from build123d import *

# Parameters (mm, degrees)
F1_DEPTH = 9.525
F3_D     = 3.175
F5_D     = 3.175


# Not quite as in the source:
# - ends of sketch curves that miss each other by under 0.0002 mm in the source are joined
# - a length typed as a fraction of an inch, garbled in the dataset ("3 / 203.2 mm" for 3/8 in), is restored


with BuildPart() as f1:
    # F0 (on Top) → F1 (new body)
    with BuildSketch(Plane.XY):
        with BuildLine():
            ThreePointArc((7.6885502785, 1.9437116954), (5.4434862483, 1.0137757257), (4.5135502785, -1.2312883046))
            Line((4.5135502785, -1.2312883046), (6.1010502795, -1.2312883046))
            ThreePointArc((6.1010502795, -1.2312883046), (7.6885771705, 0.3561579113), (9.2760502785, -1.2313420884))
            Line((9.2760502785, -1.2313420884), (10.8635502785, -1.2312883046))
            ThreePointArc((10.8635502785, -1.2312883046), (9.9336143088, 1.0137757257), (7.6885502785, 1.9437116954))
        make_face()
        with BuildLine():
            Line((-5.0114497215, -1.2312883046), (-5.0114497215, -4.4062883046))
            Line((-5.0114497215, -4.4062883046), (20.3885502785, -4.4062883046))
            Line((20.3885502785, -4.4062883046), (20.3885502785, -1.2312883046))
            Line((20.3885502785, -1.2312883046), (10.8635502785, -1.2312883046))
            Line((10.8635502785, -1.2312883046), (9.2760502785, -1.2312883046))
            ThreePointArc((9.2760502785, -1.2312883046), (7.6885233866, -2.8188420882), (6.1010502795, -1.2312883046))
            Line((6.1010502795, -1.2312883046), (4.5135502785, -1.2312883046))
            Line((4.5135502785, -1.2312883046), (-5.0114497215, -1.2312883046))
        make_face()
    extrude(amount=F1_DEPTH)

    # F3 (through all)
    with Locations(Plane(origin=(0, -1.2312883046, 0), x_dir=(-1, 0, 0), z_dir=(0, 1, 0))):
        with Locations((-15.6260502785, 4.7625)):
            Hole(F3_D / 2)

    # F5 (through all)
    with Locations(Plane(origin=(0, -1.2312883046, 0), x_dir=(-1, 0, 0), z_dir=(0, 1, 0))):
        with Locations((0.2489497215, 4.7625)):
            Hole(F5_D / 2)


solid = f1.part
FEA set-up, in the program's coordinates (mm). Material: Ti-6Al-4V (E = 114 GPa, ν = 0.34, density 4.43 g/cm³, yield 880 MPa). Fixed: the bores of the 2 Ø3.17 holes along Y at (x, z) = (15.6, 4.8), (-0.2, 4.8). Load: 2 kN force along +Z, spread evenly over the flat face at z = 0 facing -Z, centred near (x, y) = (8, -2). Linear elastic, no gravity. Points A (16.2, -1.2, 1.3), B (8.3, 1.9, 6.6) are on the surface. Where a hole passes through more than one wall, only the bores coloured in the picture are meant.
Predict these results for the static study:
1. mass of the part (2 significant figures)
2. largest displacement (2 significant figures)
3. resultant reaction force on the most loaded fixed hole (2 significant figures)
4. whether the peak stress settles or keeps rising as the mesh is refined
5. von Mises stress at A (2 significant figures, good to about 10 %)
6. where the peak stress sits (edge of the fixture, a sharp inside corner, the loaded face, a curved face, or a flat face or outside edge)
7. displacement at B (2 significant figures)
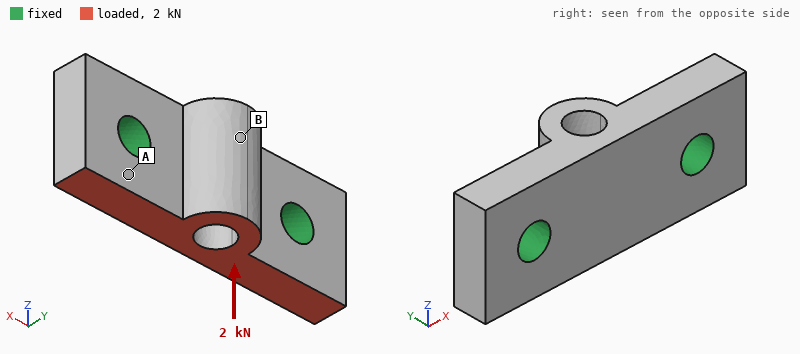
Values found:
3.5 g
6.7 µm
1.0 kN
keeps rising
29 MPa
edge of the fixture
5.1 µm
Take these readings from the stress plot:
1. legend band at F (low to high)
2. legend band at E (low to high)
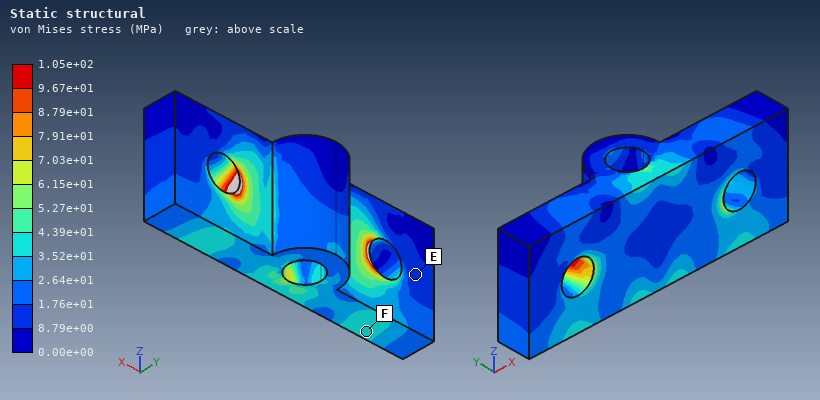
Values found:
3.52e+01 to 4.39e+01 MPa
8.79e+00 to 1.76e+01 MPa
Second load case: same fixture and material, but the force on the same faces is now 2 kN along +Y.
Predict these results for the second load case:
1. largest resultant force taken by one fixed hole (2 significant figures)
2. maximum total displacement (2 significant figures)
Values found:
1.0 kN
24 µm
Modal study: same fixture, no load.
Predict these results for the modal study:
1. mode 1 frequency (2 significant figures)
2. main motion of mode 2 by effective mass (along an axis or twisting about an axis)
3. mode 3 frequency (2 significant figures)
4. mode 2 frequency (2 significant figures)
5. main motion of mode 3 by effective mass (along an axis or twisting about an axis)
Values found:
49 kHz
along Y
71 kHz
56 kHz
along Z
